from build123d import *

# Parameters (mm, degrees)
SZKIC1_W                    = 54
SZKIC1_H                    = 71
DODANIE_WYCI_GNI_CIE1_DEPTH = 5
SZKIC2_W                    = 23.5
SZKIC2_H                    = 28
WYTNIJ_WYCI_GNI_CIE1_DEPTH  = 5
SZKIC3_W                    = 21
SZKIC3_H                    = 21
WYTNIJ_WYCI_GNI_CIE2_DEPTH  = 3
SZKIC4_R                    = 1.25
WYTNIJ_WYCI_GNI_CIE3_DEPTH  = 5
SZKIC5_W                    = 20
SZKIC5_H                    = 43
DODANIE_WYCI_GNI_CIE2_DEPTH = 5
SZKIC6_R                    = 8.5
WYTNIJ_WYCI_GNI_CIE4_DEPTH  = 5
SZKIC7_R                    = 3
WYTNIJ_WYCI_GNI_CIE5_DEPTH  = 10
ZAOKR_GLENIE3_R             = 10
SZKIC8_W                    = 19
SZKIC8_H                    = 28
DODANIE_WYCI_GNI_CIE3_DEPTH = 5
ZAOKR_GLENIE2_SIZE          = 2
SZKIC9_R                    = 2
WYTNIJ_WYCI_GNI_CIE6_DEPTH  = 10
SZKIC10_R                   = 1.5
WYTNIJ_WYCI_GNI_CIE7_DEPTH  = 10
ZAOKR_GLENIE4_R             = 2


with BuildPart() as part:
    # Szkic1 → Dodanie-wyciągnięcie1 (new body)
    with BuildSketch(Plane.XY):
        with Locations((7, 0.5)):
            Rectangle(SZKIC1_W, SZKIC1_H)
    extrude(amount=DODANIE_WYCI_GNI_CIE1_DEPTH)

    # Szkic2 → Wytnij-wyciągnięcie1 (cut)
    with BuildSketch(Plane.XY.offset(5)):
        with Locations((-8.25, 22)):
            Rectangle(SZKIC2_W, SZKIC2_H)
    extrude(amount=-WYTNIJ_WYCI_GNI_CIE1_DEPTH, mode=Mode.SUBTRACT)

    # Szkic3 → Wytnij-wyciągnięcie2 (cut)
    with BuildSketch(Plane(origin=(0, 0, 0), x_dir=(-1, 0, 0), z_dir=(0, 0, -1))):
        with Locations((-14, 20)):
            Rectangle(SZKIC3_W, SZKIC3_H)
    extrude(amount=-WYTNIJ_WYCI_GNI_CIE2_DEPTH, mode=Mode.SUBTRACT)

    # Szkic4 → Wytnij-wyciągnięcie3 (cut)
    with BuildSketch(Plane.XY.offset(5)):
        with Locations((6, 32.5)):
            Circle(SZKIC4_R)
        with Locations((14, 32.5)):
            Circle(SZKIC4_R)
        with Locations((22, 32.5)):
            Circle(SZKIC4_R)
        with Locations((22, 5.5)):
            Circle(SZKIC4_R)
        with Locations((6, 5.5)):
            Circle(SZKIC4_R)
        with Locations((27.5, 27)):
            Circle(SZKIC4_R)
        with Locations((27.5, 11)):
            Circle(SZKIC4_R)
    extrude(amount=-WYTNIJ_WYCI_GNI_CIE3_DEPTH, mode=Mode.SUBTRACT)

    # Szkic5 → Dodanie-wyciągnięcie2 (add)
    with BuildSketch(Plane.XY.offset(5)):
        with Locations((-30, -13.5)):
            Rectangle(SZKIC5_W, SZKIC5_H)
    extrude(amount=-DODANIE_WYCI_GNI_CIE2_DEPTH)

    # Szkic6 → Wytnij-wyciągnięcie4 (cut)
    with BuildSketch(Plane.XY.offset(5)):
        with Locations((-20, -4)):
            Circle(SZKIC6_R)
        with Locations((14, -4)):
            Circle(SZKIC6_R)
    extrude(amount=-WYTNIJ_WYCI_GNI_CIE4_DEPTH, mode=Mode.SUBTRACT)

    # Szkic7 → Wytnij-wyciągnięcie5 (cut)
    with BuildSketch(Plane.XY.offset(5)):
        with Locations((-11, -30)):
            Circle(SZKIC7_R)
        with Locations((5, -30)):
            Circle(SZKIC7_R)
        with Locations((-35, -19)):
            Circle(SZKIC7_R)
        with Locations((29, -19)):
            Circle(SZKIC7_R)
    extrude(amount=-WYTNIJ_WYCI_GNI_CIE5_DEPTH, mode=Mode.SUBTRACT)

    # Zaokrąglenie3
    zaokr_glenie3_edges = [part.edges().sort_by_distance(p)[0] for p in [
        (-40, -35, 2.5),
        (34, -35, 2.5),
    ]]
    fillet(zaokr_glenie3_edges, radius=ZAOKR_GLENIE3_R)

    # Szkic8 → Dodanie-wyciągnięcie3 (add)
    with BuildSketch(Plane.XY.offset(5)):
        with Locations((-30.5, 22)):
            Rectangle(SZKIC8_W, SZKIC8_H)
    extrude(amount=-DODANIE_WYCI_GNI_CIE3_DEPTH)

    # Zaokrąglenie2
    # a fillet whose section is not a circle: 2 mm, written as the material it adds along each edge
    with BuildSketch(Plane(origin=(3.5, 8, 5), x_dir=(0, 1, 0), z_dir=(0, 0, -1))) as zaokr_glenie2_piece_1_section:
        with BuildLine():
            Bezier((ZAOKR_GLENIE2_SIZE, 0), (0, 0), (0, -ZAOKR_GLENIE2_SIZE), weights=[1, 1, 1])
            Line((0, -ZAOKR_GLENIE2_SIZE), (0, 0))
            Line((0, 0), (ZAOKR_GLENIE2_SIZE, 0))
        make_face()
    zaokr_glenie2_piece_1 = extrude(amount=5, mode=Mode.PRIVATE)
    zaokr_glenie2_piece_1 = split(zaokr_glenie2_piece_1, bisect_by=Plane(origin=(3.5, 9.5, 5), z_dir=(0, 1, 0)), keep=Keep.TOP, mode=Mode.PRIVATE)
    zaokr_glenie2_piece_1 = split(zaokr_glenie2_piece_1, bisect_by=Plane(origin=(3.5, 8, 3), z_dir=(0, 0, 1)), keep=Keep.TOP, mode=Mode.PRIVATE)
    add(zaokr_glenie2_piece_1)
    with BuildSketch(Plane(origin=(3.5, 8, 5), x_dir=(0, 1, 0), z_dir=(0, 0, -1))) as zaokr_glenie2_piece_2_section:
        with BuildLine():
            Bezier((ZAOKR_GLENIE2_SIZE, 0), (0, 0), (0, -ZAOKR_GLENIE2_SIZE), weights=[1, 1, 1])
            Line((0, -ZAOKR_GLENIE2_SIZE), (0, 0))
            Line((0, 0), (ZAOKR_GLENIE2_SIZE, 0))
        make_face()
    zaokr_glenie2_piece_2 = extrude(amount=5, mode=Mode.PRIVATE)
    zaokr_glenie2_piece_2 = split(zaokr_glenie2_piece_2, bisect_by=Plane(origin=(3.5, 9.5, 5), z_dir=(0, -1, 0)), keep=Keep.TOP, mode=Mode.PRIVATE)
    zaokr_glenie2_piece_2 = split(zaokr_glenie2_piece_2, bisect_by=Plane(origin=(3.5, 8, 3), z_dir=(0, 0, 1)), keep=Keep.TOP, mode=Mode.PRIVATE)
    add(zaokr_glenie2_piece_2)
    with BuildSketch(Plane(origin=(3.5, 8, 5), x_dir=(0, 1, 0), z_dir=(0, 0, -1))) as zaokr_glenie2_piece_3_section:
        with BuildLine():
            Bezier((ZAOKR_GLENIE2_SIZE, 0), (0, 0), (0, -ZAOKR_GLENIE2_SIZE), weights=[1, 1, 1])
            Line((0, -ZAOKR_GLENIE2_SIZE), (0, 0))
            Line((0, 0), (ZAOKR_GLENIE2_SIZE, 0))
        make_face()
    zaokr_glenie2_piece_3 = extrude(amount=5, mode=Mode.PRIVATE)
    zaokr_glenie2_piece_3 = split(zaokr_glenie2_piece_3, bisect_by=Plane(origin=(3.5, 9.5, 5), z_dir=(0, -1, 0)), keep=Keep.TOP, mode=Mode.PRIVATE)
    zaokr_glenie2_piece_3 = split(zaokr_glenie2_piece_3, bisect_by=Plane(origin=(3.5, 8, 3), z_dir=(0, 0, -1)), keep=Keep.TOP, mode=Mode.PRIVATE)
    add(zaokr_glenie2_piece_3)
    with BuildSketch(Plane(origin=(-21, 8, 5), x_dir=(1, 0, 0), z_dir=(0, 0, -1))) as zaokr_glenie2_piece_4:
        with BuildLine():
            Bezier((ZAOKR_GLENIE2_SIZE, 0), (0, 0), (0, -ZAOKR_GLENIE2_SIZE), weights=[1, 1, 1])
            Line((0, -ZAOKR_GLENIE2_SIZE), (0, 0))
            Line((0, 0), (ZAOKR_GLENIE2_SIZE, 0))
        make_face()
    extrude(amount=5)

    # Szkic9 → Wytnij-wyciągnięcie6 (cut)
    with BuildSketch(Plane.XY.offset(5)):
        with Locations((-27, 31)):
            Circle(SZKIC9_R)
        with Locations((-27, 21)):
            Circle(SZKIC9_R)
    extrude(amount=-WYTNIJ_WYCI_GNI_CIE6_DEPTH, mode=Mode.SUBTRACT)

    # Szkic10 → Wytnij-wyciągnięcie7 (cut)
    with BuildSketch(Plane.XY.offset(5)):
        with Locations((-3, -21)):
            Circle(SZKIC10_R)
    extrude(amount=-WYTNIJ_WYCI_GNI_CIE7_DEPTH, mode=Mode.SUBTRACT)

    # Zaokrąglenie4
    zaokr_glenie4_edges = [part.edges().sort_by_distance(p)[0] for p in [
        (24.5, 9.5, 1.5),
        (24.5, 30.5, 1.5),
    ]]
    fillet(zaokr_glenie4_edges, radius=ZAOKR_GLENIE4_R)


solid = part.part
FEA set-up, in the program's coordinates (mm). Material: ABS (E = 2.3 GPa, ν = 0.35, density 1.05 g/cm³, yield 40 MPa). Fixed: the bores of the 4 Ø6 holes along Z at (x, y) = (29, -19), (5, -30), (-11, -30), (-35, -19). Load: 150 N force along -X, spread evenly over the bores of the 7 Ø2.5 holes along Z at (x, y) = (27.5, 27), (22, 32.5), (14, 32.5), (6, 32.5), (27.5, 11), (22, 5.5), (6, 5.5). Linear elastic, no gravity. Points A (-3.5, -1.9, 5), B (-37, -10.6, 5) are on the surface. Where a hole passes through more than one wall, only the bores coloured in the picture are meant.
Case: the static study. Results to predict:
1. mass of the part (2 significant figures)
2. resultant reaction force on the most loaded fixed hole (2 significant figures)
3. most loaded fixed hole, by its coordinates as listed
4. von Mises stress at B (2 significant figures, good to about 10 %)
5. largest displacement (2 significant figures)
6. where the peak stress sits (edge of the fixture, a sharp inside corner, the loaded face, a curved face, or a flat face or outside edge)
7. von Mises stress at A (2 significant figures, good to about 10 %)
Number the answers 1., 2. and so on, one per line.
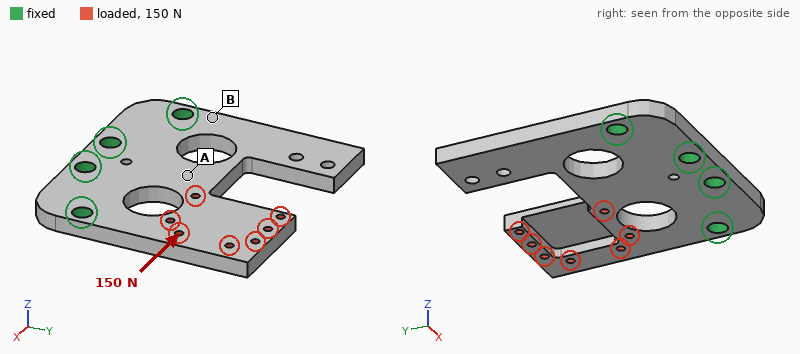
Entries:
1. 19 g
2. 140 N
3. (29, -19)
4. 0.95 MPa
5. 0.40 mm
6. a curved face
7. 2.9 MPa
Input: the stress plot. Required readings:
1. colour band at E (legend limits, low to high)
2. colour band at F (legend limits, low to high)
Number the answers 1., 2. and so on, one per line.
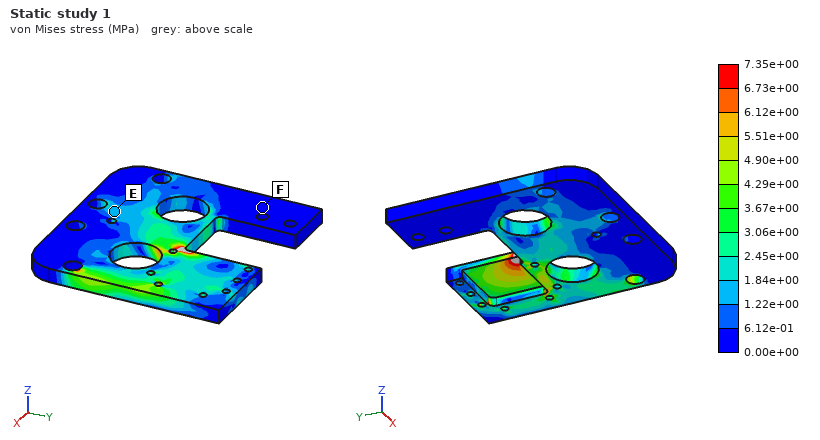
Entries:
1. 1.22e+00 to 1.84e+00 MPa
2. 0.00e+00 to 6.12e-01 MPa
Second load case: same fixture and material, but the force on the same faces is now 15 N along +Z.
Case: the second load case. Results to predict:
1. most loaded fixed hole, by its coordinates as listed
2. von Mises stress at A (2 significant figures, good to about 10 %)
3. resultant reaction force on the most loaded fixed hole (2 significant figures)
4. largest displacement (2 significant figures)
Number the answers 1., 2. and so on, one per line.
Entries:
1. (29, -19)
2. 2.0 MPa
3. 14 N
4. 1.0 mm
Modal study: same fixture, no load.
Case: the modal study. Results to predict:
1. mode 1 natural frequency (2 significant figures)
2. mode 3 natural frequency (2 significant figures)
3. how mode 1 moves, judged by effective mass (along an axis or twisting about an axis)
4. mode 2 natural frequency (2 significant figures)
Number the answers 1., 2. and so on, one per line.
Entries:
1. 400 Hz
2. 1200 Hz
3. along Z
4. 460 Hz
